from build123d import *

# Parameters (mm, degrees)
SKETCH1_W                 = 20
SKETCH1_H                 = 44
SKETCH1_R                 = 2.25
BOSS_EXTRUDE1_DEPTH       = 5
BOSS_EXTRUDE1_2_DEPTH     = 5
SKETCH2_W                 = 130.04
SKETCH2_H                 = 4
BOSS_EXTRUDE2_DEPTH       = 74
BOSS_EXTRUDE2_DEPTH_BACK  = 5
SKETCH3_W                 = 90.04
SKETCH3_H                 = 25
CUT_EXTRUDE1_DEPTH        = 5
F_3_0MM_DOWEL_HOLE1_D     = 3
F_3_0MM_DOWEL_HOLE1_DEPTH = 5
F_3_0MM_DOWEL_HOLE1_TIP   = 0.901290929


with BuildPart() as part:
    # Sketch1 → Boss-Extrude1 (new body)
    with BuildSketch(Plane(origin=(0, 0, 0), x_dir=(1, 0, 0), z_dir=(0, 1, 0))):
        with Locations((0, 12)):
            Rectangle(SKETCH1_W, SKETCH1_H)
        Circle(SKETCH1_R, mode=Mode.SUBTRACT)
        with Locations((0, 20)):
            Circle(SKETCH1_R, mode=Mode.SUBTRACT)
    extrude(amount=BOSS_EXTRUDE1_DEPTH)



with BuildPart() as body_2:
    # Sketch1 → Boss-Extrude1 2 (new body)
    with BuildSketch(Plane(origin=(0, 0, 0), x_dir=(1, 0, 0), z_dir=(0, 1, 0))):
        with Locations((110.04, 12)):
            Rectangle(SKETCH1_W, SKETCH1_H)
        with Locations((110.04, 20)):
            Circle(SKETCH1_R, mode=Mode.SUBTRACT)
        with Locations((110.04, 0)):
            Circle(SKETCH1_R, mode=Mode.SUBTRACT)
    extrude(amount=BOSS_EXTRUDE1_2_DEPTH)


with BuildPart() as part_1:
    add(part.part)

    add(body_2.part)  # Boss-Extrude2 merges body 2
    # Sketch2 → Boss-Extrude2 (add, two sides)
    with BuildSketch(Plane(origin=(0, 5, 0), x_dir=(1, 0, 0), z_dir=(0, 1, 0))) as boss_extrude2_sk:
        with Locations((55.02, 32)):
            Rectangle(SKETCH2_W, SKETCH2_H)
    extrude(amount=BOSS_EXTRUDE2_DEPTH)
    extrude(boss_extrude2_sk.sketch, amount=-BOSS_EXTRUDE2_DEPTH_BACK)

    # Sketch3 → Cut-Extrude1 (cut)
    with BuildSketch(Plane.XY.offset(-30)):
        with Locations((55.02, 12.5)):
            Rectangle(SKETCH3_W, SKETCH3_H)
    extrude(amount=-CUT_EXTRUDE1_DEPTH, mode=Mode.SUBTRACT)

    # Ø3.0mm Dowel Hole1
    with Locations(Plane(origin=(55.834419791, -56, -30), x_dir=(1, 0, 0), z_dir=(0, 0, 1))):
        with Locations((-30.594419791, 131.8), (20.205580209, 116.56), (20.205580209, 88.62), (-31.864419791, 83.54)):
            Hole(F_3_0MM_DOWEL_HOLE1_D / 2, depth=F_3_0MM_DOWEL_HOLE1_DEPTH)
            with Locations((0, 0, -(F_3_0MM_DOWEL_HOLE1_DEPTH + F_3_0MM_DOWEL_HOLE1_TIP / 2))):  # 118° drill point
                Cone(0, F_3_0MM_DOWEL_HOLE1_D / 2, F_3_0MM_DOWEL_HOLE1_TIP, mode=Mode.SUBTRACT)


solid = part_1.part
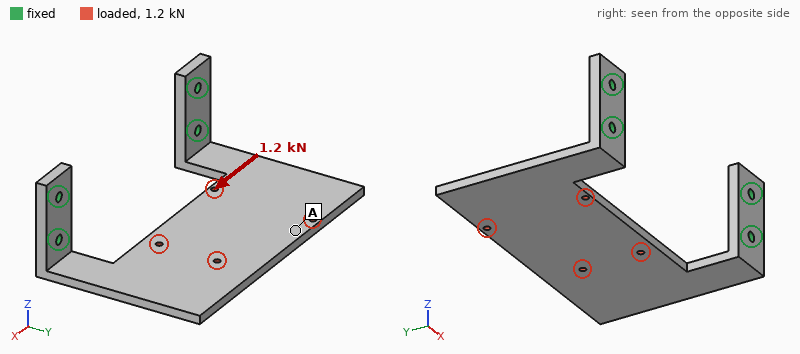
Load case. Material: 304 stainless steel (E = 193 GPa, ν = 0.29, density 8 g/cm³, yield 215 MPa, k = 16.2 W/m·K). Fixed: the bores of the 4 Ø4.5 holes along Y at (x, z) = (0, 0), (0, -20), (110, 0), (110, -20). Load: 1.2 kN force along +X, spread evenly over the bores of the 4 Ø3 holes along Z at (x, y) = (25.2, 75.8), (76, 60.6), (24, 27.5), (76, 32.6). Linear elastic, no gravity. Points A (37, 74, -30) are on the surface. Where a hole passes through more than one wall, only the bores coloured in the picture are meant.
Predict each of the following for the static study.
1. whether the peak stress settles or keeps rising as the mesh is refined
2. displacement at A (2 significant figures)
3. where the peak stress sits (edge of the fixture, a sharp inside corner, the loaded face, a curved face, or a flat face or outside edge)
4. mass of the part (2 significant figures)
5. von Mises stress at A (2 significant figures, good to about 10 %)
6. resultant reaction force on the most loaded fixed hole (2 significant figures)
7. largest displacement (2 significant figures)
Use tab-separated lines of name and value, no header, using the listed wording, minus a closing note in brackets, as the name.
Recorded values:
whether the peak stress settles or keeps rising as the mesh is refined	keeps rising
displacement at A	28 µm
where the peak stress sits	edge of the fixture
mass of the part	320 g
von Mises stress at A	6.1 MPa
resultant reaction force on the most loaded fixed hole	960 N
largest displacement	38 µm
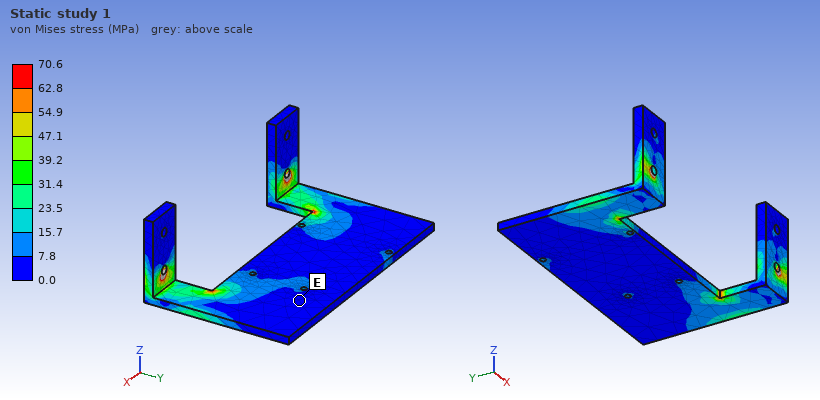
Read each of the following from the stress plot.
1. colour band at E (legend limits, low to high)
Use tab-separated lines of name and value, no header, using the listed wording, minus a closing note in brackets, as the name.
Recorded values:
colour band at E	0.0 to 7.8 MPa
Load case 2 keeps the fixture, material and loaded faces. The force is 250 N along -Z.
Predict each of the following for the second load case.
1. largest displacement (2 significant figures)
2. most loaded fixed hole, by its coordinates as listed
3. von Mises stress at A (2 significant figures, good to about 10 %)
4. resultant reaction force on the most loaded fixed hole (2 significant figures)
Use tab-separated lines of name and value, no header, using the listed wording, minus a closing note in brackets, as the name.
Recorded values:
largest displacement	0.55 mm
most loaded fixed hole, by its coordinates as listed	(0, -20)
von Mises stress at A	16 MPa
resultant reaction force on the most loaded fixed hole	150 N
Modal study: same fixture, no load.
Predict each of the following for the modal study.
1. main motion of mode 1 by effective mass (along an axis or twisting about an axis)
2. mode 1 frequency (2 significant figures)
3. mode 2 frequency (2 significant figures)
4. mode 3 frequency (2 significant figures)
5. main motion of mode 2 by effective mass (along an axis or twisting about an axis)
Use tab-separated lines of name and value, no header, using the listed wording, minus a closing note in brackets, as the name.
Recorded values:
main motion of mode 1 by effective mass	along Z
mode 1 frequency	270 Hz
mode 2 frequency	760 Hz
mode 3 frequency	1400 Hz
main motion of mode 2 by effective mass	twisting about Y
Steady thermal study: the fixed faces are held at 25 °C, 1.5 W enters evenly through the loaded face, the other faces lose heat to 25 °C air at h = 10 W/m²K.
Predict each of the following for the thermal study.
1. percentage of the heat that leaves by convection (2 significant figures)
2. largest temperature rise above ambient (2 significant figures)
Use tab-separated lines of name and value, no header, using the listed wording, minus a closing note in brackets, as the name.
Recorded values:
percentage of the heat that leaves by convection	78 %
largest temperature rise above ambient	11 K
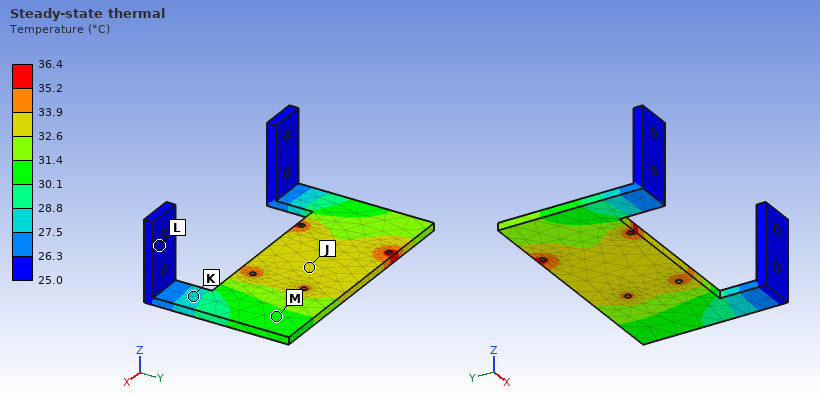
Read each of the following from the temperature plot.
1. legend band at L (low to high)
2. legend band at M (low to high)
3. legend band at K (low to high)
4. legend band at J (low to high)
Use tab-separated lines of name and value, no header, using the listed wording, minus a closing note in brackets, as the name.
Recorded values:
legend band at L	25.0 to 26.3 °C
legend band at M	30.1 to 31.4 °C
legend band at K	27.5 to 28.8 °C
legend band at J	32.6 to 33.9 °C
